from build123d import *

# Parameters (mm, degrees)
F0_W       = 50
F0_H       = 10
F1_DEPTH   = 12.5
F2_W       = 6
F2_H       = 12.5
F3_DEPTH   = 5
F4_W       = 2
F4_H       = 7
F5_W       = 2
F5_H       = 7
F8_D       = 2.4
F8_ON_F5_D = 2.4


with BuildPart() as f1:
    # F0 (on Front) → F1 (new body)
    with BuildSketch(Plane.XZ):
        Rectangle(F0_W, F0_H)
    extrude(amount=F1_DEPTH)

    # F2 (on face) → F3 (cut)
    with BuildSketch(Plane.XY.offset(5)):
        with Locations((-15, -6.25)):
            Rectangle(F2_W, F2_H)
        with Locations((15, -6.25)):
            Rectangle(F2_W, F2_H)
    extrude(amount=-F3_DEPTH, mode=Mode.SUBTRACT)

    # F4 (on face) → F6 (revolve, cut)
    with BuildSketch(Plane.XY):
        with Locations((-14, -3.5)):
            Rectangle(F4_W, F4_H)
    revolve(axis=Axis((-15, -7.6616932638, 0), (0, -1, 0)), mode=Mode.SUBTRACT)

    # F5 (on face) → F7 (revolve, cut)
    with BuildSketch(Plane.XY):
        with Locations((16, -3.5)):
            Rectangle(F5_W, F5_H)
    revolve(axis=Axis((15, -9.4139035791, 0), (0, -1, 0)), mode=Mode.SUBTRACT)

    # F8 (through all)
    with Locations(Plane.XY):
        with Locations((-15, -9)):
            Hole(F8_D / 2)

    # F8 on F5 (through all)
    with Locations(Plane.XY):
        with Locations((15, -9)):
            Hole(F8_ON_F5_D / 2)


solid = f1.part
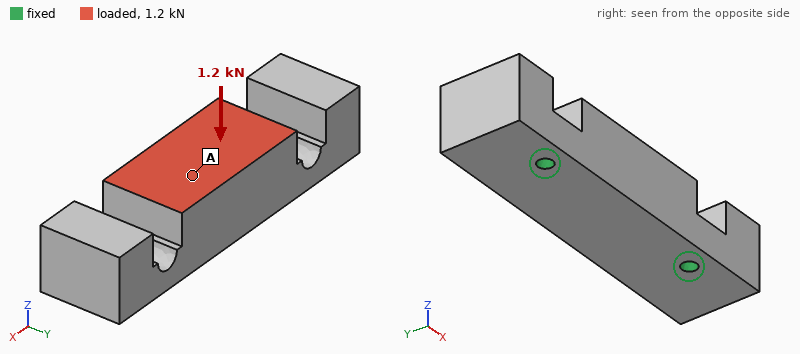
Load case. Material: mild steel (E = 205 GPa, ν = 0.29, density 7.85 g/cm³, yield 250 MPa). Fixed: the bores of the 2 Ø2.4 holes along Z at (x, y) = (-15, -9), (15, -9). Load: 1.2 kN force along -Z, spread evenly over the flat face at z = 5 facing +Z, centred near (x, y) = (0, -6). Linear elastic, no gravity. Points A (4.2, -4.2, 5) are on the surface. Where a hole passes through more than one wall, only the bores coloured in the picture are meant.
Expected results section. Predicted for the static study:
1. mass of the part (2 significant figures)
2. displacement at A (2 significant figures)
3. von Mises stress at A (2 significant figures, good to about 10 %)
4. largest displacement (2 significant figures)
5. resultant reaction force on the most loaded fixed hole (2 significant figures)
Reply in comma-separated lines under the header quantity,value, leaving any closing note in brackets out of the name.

quantity,value
mass of the part,42 g
displacement at A,4.3 µm
von Mises stress at A,13 MPa
largest displacement,5.7 µm
resultant reaction force on the most loaded fixed hole,660 N
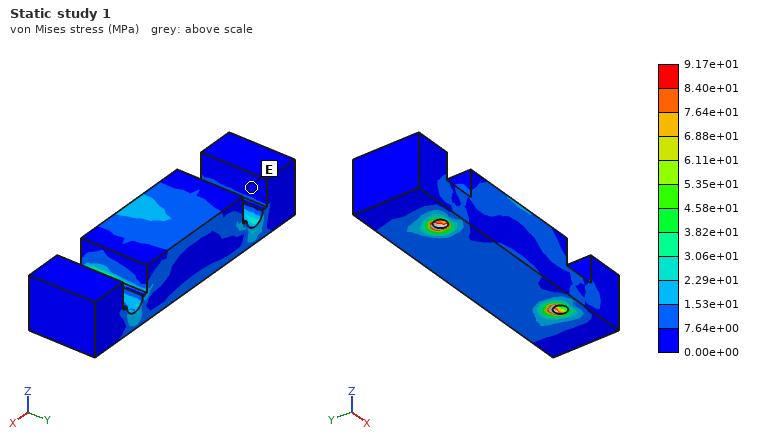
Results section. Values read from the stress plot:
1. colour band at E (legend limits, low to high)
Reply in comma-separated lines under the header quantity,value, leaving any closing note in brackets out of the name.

quantity,value
colour band at E,0.00e+00 to 7.64e+00 MPa
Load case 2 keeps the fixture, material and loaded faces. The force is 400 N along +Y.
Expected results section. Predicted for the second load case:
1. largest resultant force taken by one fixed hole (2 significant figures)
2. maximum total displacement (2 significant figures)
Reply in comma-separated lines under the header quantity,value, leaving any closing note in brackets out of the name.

quantity,value
largest resultant force taken by one fixed hole,220 N
maximum total displacement,4.6 µm
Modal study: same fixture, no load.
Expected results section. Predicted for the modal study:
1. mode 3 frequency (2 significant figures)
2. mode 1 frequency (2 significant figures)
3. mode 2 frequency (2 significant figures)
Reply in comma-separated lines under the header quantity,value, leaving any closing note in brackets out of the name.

quantity,value
mode 3 frequency,17 kHz
mode 1 frequency,14 kHz
mode 2 frequency,16 kHz
